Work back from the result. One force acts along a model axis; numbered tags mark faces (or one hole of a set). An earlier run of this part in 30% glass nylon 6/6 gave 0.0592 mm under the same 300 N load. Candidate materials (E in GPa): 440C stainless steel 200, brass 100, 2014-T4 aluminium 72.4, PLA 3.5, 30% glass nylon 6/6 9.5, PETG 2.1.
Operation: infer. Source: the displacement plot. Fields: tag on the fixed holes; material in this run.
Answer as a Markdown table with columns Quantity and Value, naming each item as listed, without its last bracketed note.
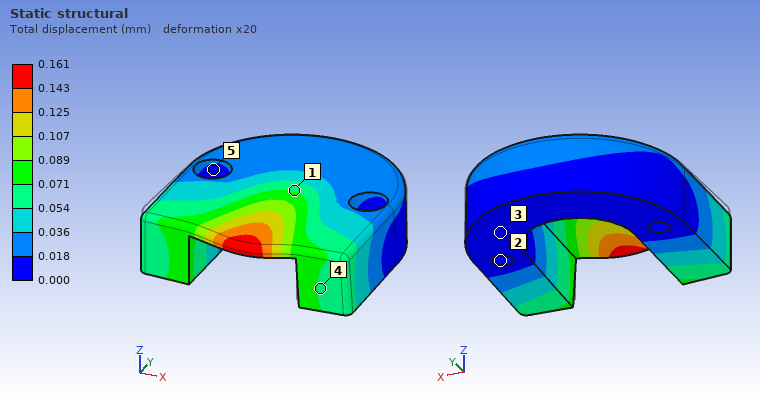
| Quantity | Value |
|---|---|
| tag on the fixed holes | 2 |
| material in this run | PLA |
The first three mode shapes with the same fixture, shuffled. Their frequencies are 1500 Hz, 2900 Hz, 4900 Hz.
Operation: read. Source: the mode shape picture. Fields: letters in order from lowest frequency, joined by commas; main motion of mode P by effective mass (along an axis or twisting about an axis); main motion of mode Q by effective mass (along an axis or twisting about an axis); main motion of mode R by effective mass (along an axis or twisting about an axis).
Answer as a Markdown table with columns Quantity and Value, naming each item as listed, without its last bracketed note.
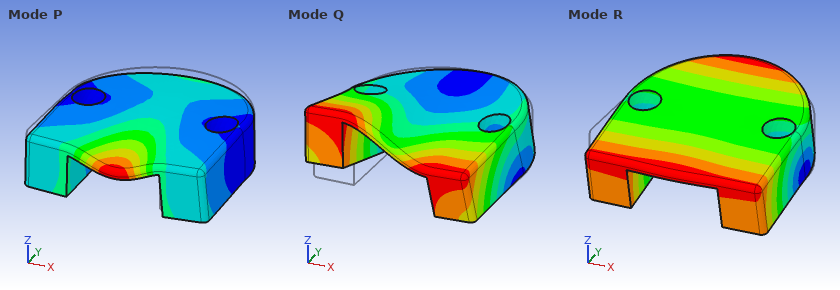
| Quantity | Value |
|---|---|
| letters in order from lowest frequency, joined by commas | R, Q, P |
| main motion of mode P by effective mass | along Z |
| main motion of mode Q by effective mass | along X |
| main motion of mode R by effective mass | along Y |
